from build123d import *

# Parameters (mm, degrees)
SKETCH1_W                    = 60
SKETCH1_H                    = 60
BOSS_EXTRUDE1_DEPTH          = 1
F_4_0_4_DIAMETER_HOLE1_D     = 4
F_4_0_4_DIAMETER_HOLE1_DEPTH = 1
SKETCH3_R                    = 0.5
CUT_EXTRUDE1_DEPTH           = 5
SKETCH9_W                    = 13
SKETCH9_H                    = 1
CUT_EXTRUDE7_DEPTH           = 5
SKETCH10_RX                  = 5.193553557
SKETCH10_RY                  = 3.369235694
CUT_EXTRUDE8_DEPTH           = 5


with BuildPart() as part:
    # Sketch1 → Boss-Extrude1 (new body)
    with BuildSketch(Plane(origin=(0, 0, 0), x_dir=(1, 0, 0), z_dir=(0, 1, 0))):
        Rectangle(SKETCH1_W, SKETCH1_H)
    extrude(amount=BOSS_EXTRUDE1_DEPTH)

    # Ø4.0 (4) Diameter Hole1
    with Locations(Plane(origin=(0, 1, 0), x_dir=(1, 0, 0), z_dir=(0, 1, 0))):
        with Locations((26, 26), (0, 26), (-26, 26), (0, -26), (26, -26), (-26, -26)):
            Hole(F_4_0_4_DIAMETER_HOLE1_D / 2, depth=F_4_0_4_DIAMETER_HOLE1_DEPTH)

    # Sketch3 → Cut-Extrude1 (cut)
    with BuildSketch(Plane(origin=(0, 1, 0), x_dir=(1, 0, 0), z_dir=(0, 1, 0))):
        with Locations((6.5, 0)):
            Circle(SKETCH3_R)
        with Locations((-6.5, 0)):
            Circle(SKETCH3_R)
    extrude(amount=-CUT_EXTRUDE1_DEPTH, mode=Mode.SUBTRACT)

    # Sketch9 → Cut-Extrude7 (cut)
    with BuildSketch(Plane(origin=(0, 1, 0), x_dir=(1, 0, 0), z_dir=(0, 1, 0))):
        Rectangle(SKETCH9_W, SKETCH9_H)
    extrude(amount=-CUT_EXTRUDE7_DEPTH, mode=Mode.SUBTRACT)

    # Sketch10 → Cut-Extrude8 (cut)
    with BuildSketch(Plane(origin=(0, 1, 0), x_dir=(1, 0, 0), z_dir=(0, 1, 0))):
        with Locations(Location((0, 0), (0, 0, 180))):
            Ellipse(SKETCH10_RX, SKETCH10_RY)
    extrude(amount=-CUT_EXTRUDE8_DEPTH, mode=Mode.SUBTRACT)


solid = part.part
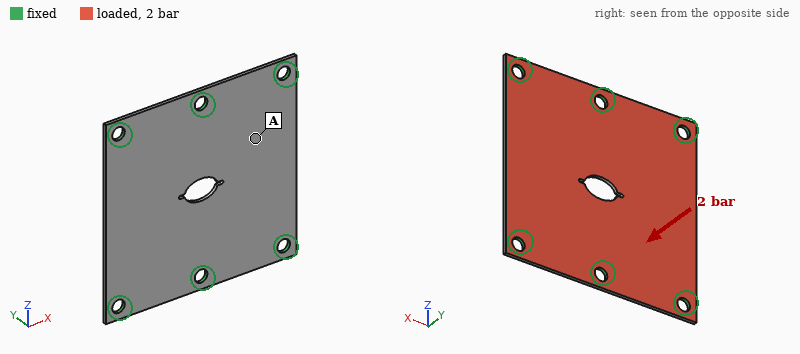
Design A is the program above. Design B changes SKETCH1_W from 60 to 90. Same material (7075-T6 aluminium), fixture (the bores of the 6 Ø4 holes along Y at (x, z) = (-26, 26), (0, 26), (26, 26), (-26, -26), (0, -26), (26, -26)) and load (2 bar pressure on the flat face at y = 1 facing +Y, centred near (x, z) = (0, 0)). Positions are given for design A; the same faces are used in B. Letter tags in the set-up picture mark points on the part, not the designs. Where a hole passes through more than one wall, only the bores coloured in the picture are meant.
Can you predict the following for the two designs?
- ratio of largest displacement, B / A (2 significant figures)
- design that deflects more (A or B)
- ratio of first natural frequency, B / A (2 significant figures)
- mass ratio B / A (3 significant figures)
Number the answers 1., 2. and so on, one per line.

1. 2.0
2. B
3. 0.78
4. 1.52
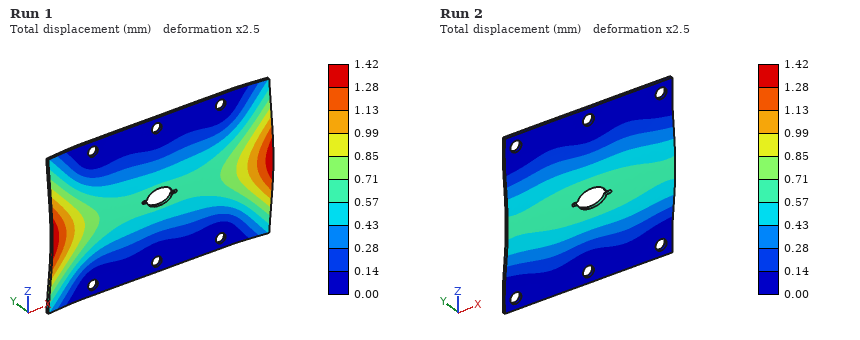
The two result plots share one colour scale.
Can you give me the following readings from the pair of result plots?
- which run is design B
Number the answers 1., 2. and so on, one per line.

1. Run 1
